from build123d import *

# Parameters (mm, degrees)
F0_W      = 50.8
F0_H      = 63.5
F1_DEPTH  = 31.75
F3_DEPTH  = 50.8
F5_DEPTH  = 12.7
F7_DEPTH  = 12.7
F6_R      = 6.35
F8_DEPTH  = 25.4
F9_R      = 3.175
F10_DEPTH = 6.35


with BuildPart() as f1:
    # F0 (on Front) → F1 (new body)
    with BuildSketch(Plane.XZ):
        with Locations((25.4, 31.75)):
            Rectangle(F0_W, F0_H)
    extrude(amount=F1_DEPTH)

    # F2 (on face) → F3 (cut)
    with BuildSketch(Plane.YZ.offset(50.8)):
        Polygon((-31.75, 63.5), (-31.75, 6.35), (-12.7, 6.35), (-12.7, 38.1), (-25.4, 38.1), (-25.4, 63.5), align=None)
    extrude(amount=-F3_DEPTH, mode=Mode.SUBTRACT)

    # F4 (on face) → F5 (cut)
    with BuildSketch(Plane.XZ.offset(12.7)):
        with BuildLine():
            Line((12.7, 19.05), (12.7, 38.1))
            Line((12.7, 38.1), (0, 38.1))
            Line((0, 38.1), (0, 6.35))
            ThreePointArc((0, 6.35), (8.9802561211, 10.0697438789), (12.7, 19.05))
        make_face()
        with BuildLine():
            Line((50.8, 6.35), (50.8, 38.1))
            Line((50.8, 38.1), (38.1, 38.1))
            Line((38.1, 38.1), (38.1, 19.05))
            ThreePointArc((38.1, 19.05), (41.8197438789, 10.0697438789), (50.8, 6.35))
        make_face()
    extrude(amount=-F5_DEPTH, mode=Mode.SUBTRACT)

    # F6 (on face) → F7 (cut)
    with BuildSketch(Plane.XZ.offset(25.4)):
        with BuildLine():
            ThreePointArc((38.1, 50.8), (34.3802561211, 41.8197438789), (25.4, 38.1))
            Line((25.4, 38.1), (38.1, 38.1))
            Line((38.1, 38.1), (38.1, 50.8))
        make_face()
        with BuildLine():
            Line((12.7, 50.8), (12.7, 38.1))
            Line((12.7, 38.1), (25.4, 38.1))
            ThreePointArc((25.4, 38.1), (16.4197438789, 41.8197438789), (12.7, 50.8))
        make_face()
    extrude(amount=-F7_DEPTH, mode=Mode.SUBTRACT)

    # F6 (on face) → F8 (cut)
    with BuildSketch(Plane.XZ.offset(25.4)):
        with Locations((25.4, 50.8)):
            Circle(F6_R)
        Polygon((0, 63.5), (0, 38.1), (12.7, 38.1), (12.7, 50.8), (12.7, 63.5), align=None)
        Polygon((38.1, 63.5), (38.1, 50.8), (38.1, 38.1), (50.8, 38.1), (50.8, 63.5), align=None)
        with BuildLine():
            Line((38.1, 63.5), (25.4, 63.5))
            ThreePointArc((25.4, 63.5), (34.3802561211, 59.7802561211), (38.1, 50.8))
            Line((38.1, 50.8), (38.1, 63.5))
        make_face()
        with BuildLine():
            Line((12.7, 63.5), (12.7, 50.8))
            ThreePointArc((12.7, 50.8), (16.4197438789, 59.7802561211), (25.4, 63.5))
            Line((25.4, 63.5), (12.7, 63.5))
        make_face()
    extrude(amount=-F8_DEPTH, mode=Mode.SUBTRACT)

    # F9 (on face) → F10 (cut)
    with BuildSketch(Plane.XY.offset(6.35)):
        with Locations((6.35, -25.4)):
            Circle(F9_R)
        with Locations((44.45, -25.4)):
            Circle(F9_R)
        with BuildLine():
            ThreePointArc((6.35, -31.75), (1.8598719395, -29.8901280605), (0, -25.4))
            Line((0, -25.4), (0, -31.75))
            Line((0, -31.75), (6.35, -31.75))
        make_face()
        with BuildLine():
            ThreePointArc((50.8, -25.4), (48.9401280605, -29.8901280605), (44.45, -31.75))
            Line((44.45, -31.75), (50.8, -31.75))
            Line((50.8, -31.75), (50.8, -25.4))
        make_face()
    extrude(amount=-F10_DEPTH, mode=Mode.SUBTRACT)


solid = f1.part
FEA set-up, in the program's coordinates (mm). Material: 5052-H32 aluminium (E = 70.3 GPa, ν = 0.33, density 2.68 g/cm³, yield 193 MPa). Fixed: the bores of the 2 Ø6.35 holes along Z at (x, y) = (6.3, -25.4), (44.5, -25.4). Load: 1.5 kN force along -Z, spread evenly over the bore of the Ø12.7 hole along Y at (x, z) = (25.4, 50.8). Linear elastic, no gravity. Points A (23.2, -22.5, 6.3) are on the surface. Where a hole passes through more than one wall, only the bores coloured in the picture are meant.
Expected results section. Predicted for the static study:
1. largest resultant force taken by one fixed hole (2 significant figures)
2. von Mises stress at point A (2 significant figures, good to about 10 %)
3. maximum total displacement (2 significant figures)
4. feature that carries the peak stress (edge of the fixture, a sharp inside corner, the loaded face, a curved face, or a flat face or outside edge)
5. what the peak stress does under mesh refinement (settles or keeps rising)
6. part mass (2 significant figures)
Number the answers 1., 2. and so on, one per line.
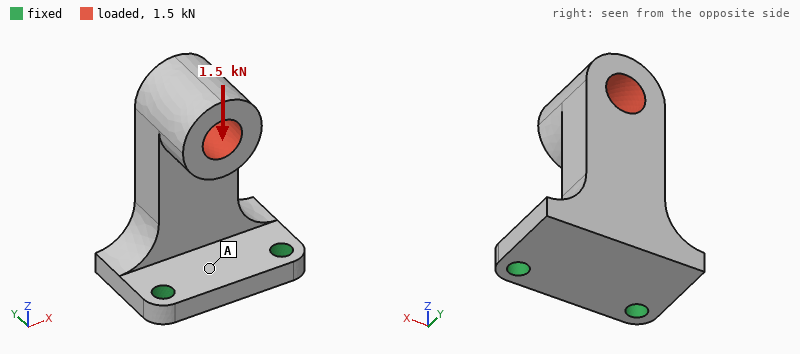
1. 750 N
2. 11 MPa
3. 62 µm
4. edge of the fixture
5. keeps rising
6. 84 g
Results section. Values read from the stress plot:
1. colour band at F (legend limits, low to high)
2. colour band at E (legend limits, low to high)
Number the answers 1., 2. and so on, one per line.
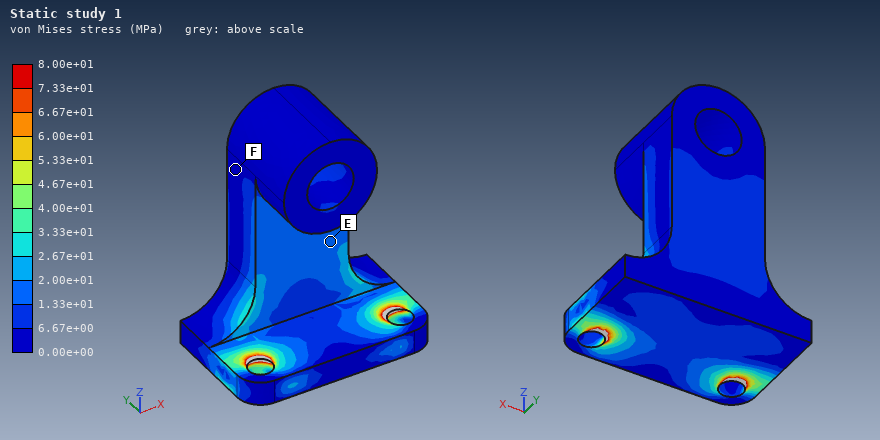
1. 0.00e+00 to 6.67e+00 MPa
2. 1.33e+01 to 2.00e+01 MPa
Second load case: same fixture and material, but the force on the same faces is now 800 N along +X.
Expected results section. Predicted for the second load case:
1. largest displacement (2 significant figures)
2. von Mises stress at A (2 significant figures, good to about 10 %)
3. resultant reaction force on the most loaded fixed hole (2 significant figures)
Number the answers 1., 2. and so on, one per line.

1. 0.12 mm
2. 19 MPa
3. 1.1 kN
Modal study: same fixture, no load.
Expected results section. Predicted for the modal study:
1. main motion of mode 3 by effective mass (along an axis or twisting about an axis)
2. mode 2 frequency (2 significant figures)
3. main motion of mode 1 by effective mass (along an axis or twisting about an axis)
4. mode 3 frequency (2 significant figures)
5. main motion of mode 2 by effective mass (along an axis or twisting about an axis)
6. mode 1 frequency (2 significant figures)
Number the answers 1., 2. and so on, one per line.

1. along Z
2. 2600 Hz
3. along Y
4. 5000 Hz
5. along X
6. 1100 Hz
